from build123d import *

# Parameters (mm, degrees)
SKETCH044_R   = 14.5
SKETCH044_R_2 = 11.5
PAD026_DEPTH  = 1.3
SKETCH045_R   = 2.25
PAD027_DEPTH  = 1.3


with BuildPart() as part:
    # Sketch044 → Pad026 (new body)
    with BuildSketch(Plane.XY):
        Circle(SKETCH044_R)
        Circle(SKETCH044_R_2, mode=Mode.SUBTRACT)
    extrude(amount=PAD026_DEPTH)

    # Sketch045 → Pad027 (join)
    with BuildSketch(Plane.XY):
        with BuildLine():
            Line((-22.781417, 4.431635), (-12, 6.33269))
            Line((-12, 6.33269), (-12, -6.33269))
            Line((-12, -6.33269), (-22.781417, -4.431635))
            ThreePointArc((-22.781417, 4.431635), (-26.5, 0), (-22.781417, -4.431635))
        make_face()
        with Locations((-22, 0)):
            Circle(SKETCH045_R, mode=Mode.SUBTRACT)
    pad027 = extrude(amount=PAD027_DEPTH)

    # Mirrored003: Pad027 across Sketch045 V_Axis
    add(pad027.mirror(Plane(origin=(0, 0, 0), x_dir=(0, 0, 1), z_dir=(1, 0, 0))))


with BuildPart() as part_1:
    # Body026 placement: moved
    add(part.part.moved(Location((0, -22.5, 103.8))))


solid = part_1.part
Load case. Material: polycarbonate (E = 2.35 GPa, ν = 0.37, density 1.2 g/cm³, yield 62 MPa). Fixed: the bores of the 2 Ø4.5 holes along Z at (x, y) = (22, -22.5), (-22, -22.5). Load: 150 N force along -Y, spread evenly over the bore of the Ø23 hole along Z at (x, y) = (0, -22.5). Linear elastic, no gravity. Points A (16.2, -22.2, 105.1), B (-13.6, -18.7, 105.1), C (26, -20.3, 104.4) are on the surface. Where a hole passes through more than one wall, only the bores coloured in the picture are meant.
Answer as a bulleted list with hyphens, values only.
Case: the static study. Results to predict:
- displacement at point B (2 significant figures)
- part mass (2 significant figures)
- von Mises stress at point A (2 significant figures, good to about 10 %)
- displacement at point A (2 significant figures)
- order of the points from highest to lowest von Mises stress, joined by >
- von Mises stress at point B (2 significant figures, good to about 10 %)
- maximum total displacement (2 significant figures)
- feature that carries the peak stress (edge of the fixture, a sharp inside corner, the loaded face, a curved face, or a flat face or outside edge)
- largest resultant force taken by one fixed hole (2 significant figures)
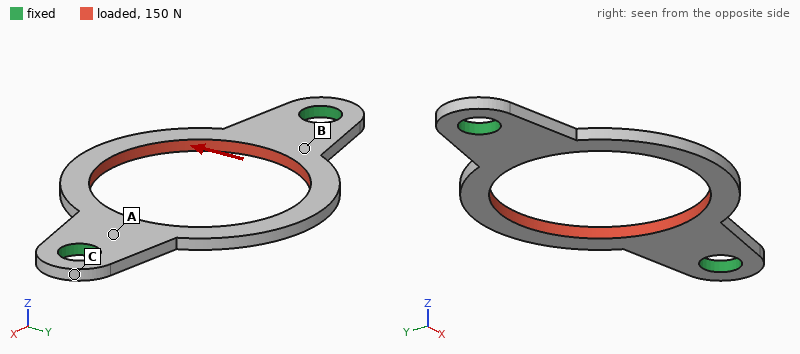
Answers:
- 0.11 mm
- 0.69 g
- 13 MPa
- 0.064 mm
- A > B > C
- 8.9 MPa
- 0.15 mm
- edge of the fixture
- 75 N
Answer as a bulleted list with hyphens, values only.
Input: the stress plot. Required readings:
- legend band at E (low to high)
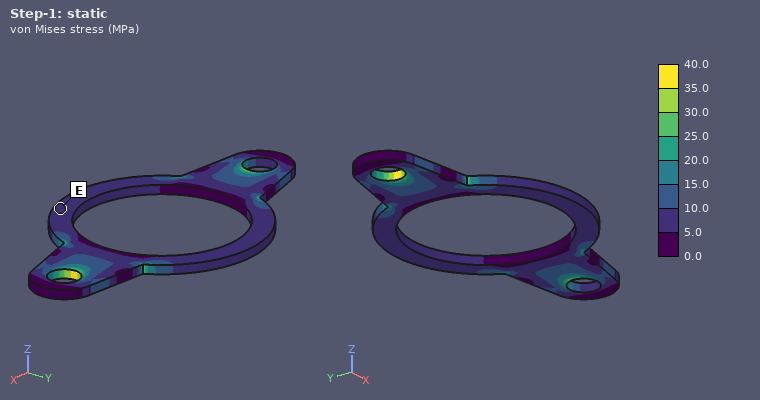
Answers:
- 5.0 to 10.0 MPa
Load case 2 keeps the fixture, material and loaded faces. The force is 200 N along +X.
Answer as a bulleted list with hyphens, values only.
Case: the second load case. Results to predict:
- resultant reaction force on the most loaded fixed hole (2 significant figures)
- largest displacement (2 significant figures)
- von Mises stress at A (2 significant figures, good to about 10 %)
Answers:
- 100 N
- 0.25 mm
- 3.4 MPa
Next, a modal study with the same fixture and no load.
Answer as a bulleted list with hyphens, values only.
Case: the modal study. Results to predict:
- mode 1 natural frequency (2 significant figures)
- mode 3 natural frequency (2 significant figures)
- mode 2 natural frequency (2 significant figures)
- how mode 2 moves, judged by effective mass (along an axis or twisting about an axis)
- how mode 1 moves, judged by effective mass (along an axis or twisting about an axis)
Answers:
- 880 Hz
- 2400 Hz
- 950 Hz
- along Z
- twisting about X
